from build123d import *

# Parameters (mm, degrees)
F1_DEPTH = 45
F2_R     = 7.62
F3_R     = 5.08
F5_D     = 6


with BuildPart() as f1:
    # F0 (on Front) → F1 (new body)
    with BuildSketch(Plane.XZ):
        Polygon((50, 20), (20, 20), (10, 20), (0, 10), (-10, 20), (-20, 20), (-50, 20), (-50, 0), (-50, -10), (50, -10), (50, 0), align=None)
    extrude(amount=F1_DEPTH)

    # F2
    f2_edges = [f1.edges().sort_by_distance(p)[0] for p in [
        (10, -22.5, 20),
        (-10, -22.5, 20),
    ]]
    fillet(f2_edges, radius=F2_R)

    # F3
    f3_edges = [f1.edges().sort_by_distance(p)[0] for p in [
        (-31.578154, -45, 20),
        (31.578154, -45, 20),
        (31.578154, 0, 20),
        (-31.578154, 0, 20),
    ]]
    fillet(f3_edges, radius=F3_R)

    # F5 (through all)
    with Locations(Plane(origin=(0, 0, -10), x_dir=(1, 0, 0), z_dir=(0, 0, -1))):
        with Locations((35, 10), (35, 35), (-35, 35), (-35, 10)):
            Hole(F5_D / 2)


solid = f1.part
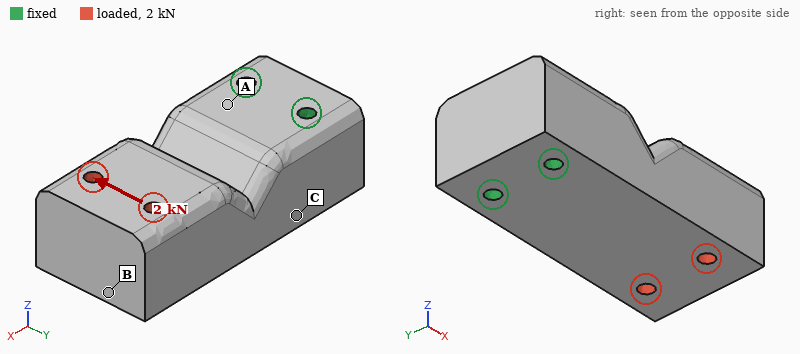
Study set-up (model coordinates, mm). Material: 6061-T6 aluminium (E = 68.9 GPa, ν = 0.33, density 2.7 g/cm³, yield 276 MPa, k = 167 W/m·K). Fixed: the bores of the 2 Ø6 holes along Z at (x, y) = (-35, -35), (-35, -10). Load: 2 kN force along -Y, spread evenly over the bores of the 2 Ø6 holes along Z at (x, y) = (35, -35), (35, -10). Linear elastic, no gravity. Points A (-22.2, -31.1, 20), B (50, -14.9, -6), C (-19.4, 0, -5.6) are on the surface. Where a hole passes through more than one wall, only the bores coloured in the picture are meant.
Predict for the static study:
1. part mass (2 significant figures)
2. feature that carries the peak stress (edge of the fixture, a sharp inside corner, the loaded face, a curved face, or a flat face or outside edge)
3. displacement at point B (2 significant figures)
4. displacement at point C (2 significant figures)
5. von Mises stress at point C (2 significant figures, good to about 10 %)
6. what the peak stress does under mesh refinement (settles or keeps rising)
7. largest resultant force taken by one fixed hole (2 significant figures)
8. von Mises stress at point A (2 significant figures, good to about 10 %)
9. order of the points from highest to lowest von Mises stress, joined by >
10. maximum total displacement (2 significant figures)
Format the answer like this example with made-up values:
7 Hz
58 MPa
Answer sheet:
340 g
edge of the fixture
30 µm
5.0 µm
12 MPa
keeps rising
5.0 kN
6.0 MPa
C > A > B
32 µm
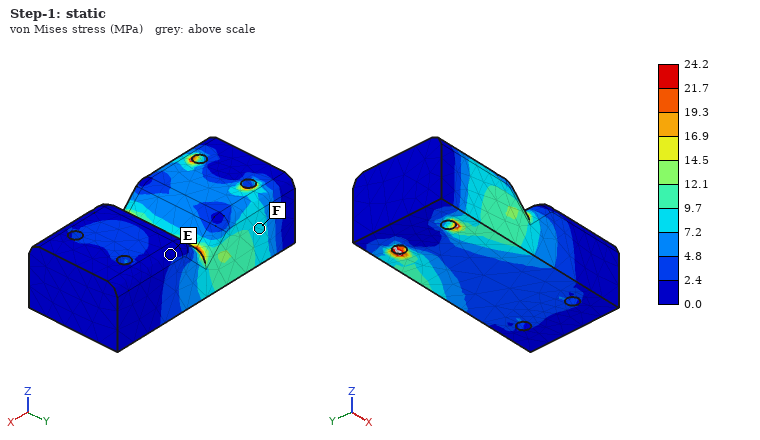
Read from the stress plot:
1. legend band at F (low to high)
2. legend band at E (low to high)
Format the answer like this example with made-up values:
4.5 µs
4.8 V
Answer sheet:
7.2 to 9.7 MPa
0.0 to 2.4 MPa
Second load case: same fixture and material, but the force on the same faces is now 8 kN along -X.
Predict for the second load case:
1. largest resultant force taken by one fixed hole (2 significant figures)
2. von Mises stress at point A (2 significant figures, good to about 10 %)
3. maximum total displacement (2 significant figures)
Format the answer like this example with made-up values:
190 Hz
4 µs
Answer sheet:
4.0 kN
5.5 MPa
19 µm
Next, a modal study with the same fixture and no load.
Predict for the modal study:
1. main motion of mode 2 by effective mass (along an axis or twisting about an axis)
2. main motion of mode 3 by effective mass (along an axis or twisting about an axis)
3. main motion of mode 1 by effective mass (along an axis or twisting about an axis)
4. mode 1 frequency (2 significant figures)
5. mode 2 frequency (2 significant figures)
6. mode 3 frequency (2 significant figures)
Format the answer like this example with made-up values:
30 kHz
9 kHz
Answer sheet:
along Y
twisting about X
along Z
2700 Hz
3900 Hz
7500 Hz
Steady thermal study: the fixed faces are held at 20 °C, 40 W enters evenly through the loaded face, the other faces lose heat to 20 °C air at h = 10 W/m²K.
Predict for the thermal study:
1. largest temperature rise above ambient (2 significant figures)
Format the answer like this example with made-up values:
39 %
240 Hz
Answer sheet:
14 K
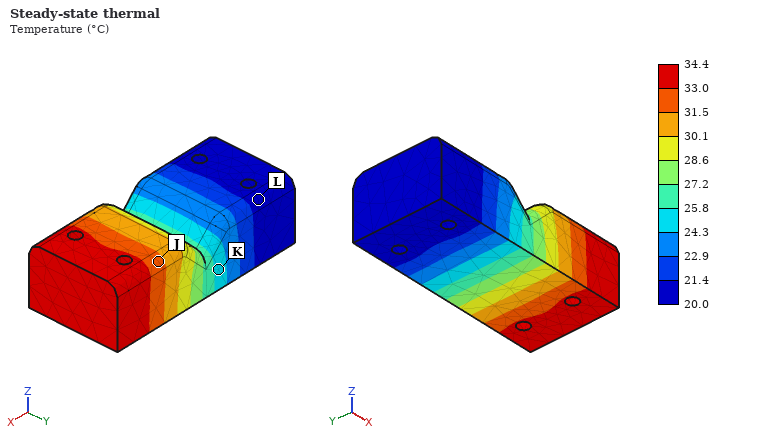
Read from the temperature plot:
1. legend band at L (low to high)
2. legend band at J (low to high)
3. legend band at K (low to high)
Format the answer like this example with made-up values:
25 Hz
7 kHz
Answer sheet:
20.0 to 21.4 °C
31.5 to 33.0 °C
24.3 to 25.8 °C
